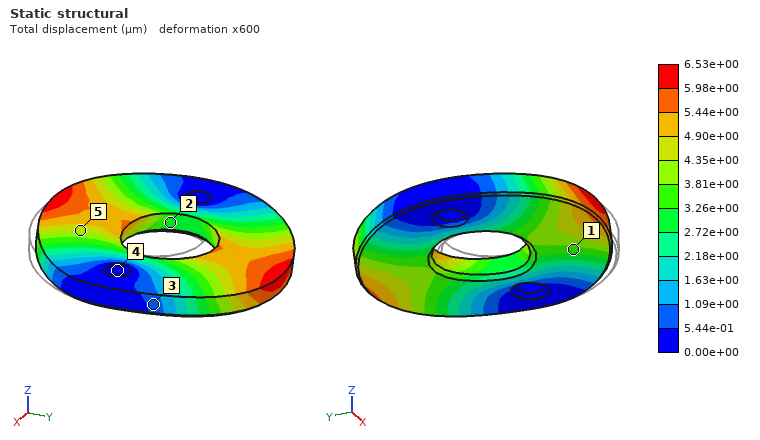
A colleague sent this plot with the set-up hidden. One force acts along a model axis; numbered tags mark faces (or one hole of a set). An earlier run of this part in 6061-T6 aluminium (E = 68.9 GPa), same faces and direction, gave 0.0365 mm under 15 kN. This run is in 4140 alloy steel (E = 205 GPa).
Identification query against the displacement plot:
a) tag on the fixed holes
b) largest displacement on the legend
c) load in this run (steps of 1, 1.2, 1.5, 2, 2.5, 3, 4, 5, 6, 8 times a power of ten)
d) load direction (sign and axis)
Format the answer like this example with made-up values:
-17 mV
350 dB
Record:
4
6.53e+00 µm
8 kN
+Y
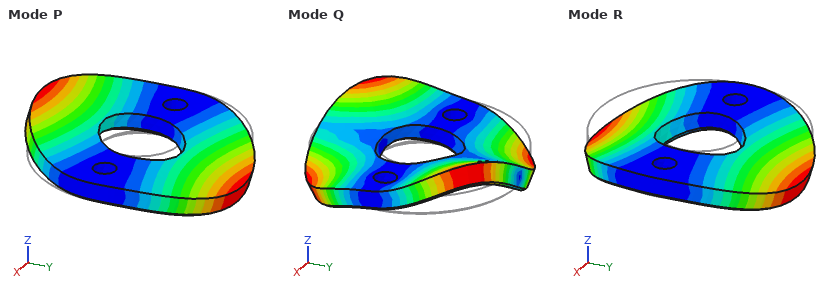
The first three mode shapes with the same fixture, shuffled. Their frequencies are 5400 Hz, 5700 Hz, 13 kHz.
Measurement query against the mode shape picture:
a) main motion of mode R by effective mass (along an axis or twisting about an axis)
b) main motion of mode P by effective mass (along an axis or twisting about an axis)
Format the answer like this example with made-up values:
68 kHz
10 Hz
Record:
along Z
twisting about X
